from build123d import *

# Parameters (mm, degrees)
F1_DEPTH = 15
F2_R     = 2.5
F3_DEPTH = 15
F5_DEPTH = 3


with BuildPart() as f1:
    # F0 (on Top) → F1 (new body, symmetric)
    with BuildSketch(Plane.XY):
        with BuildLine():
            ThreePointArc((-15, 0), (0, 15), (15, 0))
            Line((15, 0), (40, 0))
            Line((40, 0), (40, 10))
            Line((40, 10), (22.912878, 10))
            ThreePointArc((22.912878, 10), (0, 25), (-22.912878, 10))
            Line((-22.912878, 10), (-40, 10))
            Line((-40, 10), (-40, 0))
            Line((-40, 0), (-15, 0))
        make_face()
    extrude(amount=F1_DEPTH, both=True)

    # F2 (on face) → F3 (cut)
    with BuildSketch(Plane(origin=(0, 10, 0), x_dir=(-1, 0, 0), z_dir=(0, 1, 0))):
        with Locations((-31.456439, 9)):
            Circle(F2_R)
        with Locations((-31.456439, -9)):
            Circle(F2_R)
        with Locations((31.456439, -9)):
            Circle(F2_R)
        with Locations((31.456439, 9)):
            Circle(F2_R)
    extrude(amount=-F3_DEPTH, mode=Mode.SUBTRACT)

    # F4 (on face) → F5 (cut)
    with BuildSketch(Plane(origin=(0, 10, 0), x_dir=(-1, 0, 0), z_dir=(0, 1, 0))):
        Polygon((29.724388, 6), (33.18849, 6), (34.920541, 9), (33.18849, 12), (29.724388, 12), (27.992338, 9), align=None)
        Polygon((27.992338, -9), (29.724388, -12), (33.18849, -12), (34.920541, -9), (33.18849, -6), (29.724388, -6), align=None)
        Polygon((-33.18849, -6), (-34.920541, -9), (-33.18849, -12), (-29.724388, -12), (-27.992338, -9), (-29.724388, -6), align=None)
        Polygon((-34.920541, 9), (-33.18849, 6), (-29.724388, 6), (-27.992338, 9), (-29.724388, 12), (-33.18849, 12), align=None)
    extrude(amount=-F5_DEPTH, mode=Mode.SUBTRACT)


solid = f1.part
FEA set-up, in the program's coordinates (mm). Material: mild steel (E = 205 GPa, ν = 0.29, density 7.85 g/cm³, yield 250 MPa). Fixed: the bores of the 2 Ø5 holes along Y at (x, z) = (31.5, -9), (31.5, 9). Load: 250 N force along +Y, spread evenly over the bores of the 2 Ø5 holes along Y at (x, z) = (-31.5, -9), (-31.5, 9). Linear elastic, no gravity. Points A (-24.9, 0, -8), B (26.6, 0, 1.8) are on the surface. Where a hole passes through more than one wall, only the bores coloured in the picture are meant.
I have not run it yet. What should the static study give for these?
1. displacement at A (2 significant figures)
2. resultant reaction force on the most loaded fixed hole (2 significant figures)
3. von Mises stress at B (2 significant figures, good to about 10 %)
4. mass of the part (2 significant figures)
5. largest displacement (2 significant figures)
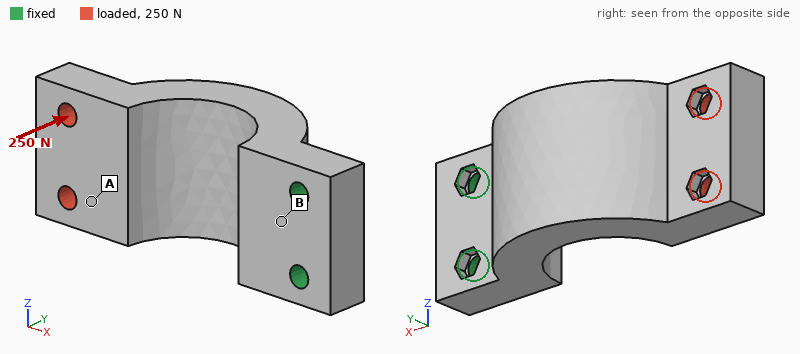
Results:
47 µm
130 N
22 MPa
210 g
65 µm
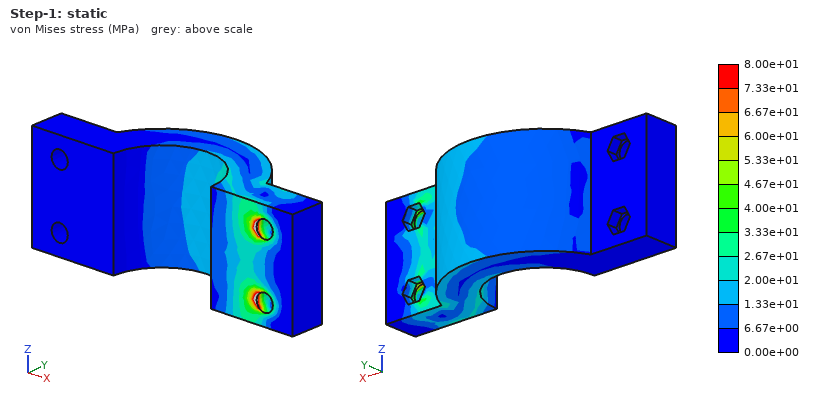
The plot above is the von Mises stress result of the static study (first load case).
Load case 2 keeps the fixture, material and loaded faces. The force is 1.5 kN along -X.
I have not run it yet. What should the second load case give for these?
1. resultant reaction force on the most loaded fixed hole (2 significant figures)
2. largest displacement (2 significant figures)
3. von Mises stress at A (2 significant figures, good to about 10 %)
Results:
750 N
77 µm
9.4 MPa
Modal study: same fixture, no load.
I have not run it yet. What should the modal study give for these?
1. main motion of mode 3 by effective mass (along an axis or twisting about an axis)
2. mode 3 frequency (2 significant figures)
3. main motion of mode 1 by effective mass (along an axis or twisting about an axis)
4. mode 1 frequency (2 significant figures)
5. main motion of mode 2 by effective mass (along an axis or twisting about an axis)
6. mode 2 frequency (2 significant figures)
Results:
along X
4900 Hz
along Y
1300 Hz
along Z
2600 Hz
